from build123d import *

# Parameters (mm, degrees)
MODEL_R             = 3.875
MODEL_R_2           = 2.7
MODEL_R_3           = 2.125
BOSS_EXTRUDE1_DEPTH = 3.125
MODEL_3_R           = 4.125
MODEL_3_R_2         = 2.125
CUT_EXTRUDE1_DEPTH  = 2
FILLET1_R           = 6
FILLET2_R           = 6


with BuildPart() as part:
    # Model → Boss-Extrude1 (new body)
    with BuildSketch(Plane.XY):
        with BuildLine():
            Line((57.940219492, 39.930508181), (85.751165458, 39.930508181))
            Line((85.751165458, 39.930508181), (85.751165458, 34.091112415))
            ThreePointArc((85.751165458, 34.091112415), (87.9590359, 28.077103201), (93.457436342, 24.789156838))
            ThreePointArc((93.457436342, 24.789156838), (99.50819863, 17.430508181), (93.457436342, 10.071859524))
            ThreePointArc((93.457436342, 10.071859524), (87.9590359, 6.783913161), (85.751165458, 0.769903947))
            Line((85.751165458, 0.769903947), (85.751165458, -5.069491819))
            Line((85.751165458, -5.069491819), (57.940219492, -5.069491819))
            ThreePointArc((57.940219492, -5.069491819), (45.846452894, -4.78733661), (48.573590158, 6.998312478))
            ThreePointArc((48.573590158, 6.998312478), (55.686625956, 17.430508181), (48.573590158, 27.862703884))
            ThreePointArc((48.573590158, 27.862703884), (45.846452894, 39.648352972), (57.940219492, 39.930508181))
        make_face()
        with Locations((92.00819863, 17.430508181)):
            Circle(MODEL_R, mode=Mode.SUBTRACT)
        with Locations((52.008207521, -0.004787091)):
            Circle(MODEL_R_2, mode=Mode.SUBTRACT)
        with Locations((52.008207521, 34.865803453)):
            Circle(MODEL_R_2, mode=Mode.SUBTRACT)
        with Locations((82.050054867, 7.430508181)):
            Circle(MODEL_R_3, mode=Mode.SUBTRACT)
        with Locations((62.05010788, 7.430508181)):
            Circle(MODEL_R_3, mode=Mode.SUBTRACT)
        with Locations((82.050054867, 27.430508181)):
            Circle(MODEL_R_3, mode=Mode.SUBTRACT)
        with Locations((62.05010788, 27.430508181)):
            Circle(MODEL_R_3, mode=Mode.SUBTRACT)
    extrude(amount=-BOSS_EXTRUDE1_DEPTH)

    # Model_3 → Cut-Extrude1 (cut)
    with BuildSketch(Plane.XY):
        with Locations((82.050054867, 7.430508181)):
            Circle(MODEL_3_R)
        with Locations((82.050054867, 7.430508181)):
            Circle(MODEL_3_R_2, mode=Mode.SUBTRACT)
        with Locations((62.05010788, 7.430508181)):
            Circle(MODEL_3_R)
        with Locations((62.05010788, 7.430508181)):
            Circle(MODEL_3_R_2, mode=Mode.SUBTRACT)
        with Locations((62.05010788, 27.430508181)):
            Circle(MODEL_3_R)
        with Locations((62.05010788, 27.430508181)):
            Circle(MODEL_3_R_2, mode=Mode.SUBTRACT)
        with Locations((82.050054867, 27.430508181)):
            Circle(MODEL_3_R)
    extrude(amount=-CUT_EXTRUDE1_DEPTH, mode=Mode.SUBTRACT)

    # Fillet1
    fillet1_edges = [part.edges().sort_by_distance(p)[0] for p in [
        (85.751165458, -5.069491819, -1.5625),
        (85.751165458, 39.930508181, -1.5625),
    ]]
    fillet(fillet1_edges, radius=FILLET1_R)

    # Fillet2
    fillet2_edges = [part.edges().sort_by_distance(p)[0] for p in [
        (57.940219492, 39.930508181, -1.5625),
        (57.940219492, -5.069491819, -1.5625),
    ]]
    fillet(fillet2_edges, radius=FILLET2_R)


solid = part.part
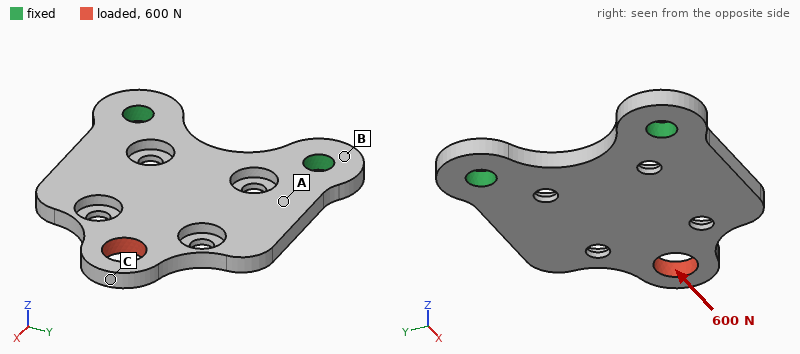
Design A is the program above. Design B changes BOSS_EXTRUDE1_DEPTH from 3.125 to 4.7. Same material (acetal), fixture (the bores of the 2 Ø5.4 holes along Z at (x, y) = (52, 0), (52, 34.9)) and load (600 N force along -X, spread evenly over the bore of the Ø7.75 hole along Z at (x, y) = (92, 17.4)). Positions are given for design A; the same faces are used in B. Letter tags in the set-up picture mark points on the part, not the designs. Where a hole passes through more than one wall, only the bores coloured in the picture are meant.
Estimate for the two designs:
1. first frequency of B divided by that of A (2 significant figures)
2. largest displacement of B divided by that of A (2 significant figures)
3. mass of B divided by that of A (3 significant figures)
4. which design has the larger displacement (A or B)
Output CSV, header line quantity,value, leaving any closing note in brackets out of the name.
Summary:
quantity,value
first frequency of B divided by that of A,1.4
largest displacement of B divided by that of A,0.50
mass of B divided by that of A,1.53
which design has the larger displacement,A
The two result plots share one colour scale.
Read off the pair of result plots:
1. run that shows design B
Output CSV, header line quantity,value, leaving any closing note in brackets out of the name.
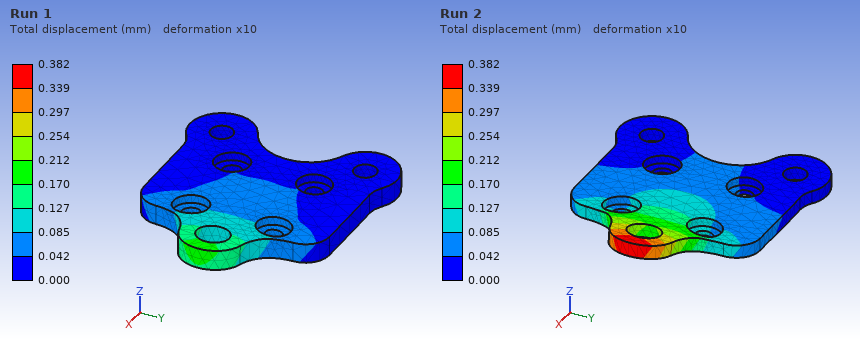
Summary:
quantity,value
run that shows design B,Run 1
